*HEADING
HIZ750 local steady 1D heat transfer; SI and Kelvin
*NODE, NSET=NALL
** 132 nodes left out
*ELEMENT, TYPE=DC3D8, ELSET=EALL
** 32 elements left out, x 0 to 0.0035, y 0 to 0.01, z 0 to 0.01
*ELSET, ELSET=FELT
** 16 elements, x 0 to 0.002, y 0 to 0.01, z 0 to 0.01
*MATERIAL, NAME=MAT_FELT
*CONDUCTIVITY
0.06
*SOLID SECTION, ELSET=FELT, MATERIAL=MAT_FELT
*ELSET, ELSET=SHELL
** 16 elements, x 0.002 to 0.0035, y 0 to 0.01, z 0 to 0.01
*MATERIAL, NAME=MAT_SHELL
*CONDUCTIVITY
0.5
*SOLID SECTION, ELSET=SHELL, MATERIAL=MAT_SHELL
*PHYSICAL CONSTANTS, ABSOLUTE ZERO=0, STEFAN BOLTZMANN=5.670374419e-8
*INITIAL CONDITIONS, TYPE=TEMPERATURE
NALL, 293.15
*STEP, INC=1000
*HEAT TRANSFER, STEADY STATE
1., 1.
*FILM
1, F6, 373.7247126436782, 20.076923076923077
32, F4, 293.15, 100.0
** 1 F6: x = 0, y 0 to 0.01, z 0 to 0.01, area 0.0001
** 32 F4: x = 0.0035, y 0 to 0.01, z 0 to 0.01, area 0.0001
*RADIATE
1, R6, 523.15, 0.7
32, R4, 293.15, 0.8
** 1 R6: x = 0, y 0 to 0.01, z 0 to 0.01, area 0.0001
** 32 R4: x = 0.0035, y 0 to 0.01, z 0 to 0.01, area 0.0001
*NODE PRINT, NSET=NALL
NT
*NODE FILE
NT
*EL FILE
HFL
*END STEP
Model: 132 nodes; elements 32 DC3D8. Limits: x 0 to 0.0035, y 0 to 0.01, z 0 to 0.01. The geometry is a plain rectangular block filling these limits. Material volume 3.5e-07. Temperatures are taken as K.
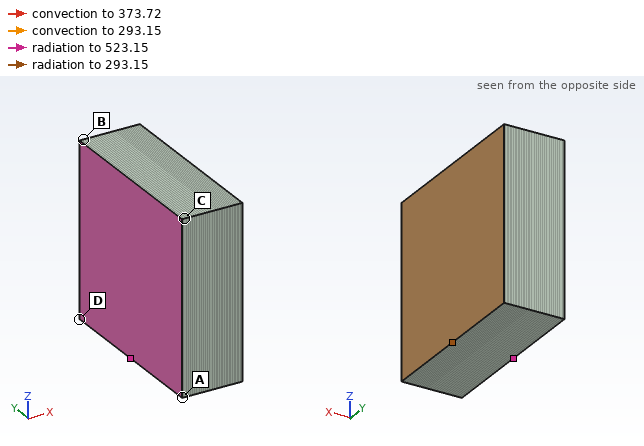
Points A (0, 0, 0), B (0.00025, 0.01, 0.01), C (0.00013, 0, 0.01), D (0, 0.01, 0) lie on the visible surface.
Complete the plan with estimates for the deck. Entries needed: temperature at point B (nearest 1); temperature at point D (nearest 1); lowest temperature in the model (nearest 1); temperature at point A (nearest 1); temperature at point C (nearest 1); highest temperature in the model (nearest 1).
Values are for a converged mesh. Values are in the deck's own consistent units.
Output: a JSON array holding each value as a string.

["374 K", "382 K", "312 K", "382 K", "378 K", "382 K"]
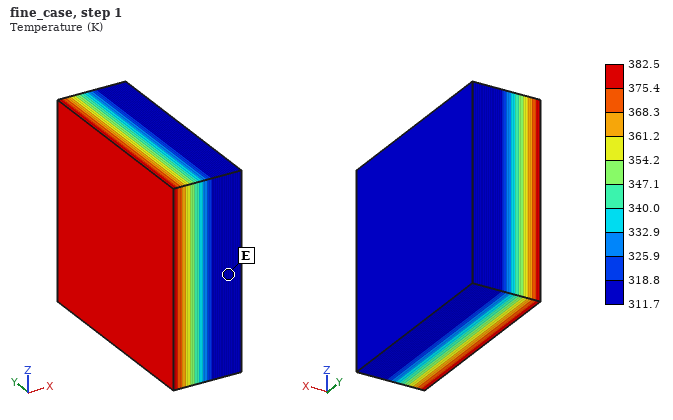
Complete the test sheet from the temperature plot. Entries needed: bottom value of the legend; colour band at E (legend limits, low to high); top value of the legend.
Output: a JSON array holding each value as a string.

["311.7 K", "311.7 to 318.8 K", "382.5 K"]
